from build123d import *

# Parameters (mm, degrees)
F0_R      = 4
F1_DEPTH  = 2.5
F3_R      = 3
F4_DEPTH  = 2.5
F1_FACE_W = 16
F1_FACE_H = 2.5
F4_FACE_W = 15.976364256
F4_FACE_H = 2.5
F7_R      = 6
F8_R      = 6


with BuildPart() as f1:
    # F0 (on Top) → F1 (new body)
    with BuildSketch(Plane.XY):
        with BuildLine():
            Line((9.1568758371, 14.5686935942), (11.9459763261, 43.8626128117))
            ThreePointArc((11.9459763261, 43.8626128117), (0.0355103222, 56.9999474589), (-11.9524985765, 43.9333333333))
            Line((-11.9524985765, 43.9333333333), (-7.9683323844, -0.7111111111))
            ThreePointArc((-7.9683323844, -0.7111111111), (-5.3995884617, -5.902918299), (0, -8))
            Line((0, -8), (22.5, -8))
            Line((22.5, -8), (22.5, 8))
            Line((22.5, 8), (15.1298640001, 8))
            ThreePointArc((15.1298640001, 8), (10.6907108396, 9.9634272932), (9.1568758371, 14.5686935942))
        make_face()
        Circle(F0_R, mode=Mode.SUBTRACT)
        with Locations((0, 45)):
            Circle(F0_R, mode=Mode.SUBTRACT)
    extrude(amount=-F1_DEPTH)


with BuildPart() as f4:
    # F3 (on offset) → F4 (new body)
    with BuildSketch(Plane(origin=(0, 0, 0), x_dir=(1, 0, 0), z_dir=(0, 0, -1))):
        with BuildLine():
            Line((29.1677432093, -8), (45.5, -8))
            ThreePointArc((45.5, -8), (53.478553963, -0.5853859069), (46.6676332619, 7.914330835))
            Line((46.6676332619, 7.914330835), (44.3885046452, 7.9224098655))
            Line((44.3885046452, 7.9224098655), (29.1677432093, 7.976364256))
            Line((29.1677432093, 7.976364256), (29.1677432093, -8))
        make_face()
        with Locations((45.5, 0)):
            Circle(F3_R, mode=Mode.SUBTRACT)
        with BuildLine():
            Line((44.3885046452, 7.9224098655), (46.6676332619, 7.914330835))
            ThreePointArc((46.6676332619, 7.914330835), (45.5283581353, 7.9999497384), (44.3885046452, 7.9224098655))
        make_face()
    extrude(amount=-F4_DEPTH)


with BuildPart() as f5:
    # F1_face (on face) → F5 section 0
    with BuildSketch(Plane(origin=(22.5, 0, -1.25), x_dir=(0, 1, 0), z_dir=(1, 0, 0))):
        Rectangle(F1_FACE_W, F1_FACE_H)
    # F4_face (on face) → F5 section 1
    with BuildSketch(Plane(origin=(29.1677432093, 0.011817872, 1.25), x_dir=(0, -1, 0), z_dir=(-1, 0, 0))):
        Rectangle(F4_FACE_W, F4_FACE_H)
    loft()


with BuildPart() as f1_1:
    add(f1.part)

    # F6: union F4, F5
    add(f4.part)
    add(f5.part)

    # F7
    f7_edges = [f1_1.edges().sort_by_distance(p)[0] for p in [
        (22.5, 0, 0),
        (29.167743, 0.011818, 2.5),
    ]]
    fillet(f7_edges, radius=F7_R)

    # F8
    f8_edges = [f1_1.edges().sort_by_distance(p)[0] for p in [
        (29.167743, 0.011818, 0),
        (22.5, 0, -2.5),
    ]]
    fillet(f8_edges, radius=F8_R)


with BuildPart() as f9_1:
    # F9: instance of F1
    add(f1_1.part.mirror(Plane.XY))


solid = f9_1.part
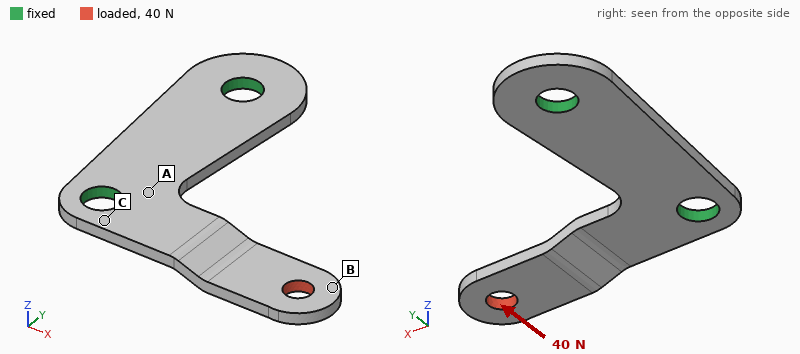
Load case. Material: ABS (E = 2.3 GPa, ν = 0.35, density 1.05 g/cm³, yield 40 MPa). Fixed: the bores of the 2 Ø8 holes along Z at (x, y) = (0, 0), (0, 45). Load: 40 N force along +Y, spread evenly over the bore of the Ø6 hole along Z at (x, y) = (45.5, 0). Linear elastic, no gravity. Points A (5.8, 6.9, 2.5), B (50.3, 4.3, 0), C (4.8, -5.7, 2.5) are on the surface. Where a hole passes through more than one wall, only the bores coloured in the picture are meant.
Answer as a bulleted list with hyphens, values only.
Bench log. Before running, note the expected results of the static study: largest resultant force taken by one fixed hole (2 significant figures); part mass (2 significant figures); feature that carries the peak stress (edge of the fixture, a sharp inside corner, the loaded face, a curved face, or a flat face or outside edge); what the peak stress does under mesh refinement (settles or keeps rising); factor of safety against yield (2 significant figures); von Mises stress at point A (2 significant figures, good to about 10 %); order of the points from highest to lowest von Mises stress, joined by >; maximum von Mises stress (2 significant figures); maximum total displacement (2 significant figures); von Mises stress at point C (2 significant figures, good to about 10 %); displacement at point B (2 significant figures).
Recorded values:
- 32 N
- 4.8 g
- a curved face
- settles
- 2.0
- 6.1 MPa
- C > A > B
- 20 MPa
- 0.85 mm
- 10 MPa
- 0.79 mm
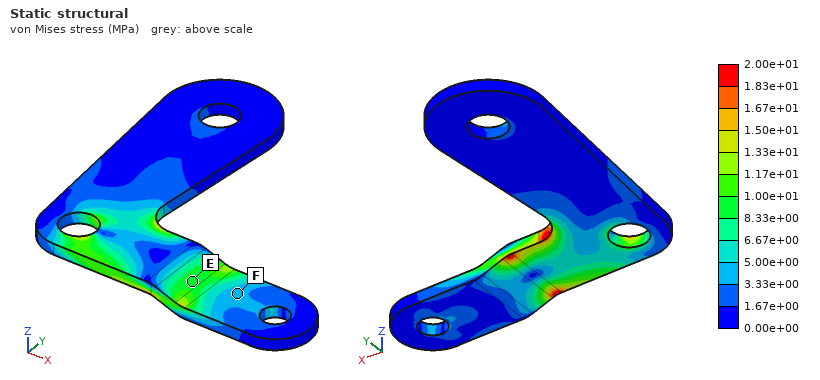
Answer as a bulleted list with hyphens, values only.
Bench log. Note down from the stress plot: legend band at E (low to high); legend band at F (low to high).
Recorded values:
- 8.33e+00 to 1.00e+01 MPa
- 3.33e+00 to 5.00e+00 MPa
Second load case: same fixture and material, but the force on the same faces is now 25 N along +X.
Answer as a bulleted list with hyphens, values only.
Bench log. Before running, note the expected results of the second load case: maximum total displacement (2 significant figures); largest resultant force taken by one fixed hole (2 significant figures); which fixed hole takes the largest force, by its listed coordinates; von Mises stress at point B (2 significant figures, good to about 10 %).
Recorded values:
- 1.1 mm
- 24 N
- (0, 0)
- 0.40 MPa
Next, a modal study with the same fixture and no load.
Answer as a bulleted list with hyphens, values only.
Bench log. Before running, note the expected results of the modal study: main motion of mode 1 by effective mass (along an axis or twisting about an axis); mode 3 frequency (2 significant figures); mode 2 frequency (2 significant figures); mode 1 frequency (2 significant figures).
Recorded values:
- along Z
- 1500 Hz
- 1400 Hz
- 280 Hz
